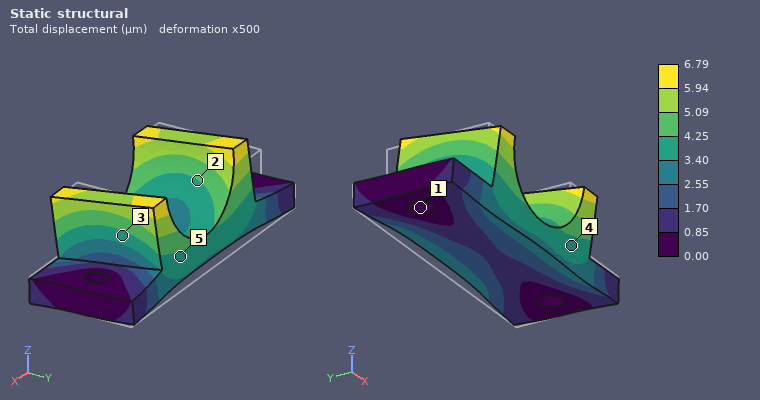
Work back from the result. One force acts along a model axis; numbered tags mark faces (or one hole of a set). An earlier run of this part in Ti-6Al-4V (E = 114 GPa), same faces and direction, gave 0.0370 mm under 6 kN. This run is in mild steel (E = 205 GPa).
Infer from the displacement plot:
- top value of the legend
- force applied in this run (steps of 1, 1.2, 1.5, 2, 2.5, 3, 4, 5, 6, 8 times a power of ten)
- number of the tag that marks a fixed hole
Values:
6.79 µm
2 kN
1
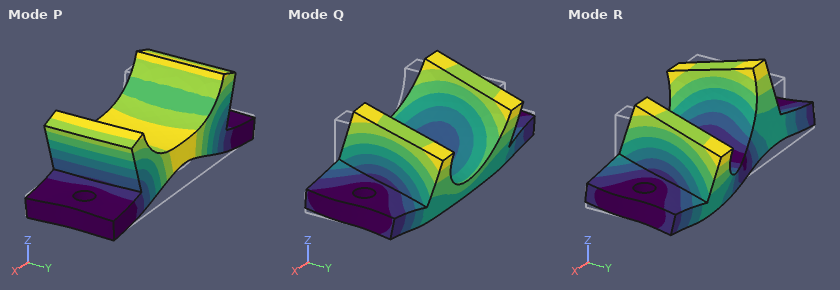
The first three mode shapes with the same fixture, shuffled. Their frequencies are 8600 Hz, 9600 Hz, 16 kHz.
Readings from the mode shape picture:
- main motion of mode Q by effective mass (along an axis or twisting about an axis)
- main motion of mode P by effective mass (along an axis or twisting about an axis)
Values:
along Y
along Z
